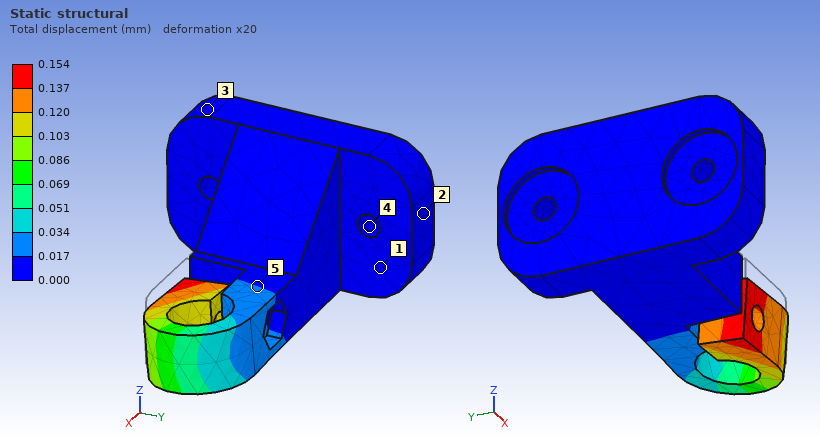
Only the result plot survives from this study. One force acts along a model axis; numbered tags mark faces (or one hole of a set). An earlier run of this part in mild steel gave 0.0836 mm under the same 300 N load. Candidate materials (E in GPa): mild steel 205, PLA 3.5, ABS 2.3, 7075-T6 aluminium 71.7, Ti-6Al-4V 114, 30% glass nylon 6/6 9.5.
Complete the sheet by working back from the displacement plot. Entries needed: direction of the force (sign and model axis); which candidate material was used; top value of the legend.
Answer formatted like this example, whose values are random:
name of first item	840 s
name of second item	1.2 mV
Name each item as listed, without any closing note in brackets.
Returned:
direction of the force	-Z
which candidate material was used	Ti-6Al-4V
top value of the legend	0.154 mm
